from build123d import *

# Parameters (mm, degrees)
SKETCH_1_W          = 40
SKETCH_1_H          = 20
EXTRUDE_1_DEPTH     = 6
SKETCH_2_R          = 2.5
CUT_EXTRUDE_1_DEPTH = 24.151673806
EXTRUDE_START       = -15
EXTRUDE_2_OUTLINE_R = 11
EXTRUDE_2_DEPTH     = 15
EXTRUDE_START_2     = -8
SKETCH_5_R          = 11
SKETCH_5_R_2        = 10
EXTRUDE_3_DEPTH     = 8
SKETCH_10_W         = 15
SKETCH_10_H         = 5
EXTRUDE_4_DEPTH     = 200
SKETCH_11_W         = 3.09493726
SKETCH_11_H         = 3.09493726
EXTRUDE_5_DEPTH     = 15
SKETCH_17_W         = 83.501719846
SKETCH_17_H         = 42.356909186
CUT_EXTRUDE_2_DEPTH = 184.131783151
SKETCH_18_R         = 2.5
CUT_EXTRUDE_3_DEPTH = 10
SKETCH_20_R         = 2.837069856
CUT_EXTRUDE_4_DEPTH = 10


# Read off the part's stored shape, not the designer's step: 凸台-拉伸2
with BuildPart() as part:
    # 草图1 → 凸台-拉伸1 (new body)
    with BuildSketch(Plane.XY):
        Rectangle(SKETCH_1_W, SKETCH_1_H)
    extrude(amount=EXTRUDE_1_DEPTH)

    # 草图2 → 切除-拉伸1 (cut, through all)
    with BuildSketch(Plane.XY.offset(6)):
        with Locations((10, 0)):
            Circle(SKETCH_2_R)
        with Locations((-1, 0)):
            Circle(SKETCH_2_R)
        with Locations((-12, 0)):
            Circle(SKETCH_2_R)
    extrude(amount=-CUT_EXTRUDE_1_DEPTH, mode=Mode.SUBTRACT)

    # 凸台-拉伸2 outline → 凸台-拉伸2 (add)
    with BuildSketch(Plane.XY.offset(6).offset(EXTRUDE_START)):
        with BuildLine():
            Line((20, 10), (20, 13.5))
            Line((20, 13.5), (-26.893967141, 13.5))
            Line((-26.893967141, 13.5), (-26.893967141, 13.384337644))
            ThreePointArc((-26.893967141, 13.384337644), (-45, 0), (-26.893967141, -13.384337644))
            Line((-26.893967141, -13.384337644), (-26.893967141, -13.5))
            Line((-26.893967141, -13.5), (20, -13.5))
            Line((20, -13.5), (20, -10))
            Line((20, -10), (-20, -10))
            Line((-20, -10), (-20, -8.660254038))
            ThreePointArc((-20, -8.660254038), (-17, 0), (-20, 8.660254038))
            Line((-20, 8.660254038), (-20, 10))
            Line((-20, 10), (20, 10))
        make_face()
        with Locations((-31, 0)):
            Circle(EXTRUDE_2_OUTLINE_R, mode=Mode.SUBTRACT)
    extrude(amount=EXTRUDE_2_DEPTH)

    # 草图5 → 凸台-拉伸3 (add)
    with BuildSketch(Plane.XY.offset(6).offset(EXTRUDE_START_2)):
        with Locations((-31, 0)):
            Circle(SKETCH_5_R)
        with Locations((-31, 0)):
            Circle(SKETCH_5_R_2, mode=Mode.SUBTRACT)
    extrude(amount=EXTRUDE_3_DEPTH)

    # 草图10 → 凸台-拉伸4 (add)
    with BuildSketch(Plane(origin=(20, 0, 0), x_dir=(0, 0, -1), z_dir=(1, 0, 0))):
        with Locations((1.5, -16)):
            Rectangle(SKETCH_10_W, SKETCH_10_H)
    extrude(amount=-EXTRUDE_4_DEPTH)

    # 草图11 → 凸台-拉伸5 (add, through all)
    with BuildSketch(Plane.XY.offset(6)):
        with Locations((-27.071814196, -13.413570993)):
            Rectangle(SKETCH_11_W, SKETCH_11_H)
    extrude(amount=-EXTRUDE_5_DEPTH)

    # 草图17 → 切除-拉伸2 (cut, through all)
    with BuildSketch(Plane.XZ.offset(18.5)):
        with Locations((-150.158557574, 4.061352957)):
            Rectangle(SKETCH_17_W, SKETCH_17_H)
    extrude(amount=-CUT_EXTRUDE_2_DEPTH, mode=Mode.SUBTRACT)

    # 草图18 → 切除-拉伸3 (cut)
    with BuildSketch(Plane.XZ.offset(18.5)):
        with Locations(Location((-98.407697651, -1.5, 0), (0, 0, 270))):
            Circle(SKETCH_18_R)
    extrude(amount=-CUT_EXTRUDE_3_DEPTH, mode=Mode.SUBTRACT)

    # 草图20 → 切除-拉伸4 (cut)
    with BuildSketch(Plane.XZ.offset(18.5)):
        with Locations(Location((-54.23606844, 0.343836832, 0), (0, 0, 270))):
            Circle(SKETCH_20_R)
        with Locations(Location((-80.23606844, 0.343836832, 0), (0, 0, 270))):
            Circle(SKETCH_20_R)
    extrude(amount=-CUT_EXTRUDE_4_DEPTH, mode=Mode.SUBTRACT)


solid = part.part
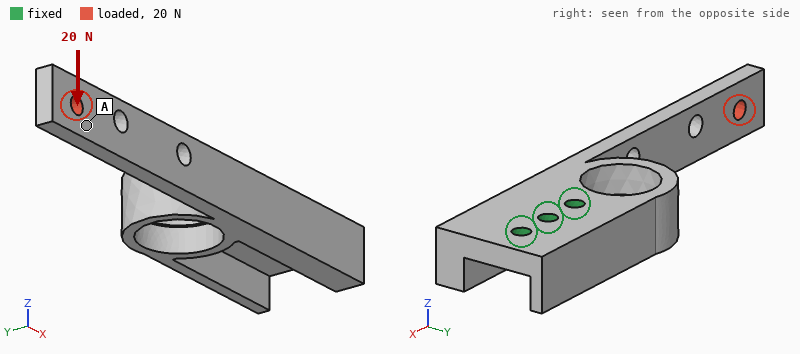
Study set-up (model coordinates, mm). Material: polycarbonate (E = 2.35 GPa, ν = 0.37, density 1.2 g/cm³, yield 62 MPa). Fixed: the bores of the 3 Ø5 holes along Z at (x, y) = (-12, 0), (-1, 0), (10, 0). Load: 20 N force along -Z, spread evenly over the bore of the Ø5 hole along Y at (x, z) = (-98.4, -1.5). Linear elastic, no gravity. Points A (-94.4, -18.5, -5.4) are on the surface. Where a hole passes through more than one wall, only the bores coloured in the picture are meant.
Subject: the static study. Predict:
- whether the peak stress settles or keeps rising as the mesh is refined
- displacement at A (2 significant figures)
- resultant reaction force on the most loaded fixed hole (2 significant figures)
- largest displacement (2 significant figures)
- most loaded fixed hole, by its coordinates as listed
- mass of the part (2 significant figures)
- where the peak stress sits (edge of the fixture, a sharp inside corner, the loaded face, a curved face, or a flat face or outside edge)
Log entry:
keeps rising
1.1 mm
81 N
1.4 mm
(-12, 0)
27 g
edge of the fixture
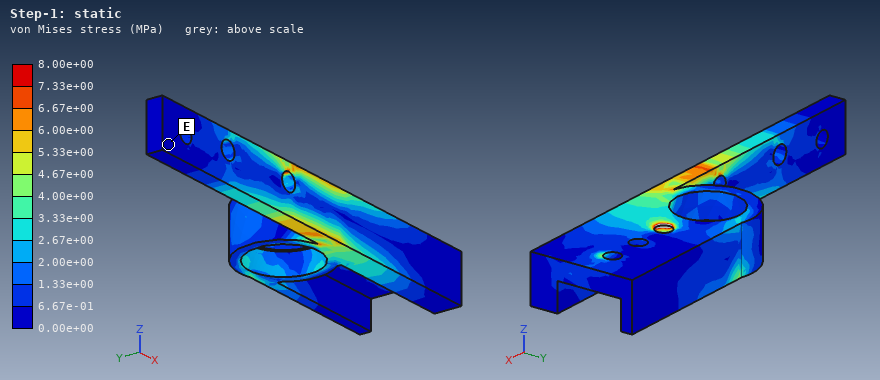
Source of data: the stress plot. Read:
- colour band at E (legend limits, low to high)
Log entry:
0.00e+00 to 6.67e-01 MPa
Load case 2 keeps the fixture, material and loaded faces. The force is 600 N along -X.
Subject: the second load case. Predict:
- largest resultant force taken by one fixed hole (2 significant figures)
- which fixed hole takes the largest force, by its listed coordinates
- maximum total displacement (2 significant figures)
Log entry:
450 N
(-12, 0)
1.1 mm
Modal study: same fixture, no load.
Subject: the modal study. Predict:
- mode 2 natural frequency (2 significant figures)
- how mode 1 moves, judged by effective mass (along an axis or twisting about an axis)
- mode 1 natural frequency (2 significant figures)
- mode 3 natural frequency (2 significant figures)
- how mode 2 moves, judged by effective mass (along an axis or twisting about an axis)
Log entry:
380 Hz
along Y
180 Hz
1100 Hz
along Z
